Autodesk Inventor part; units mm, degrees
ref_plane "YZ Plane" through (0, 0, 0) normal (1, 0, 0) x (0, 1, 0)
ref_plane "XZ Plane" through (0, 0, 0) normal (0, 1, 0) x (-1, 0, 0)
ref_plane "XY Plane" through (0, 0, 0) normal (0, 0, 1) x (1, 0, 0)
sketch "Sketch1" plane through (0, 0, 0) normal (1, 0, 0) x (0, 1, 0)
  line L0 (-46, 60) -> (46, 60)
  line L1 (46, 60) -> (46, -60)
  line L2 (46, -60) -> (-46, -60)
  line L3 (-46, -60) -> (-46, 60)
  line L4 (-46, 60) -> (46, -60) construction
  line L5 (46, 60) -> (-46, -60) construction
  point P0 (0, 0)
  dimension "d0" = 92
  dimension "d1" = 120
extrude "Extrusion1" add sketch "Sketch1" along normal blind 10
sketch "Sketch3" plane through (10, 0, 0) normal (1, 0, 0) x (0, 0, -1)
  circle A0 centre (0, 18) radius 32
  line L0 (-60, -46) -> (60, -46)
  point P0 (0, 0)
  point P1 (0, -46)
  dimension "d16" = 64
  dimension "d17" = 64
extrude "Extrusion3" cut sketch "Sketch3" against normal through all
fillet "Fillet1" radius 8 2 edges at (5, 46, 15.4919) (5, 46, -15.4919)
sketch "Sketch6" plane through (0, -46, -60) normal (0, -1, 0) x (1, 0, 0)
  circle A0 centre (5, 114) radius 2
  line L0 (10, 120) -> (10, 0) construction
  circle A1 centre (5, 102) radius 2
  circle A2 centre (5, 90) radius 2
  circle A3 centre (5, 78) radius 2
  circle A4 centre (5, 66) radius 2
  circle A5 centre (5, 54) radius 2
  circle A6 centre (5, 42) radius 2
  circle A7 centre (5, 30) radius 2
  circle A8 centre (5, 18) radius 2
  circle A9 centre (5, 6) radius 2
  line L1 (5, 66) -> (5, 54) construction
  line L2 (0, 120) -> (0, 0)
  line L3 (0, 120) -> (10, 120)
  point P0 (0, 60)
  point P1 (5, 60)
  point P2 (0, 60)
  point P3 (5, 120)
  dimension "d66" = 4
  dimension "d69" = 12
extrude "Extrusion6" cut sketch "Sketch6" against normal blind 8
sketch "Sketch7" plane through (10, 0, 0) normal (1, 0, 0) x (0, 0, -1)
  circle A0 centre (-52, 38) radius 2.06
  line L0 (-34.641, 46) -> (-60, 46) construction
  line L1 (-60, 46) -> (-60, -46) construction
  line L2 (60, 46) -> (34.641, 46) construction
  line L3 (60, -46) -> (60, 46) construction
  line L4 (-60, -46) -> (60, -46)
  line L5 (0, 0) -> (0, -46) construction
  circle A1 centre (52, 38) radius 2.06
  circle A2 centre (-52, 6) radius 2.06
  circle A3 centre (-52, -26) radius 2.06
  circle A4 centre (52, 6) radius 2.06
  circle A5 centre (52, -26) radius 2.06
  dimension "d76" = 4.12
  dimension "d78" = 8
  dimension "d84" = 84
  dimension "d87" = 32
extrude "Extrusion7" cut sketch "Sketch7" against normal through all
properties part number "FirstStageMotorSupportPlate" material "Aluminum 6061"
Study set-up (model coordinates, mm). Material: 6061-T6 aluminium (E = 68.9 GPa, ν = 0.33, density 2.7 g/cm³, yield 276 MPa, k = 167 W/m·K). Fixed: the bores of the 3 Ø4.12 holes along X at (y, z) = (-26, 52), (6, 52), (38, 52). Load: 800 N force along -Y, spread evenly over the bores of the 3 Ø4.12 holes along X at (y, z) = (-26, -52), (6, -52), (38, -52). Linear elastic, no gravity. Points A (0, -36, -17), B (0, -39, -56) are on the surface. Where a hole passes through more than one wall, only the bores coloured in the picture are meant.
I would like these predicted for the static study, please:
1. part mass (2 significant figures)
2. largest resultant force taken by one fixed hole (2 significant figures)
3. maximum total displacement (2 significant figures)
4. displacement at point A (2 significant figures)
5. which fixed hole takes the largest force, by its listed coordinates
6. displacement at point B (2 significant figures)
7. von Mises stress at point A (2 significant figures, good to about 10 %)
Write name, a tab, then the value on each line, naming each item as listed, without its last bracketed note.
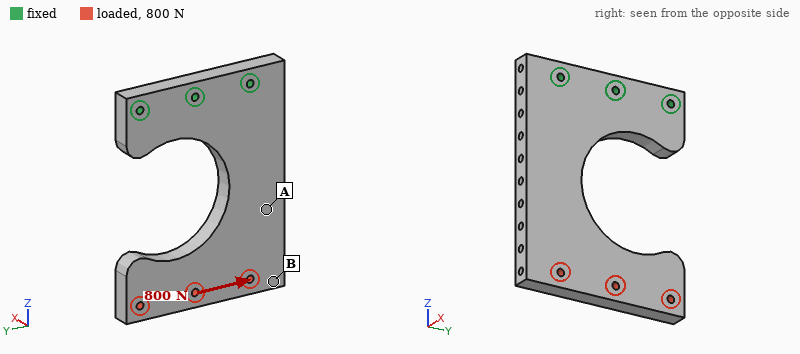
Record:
part mass	210 g
largest resultant force taken by one fixed hole	2.1 kN
maximum total displacement	0.17 mm
displacement at point A	0.055 mm
which fixed hole takes the largest force, by its listed coordinates	(-26, 52)
displacement at point B	0.12 mm
von Mises stress at point A	8.9 MPa
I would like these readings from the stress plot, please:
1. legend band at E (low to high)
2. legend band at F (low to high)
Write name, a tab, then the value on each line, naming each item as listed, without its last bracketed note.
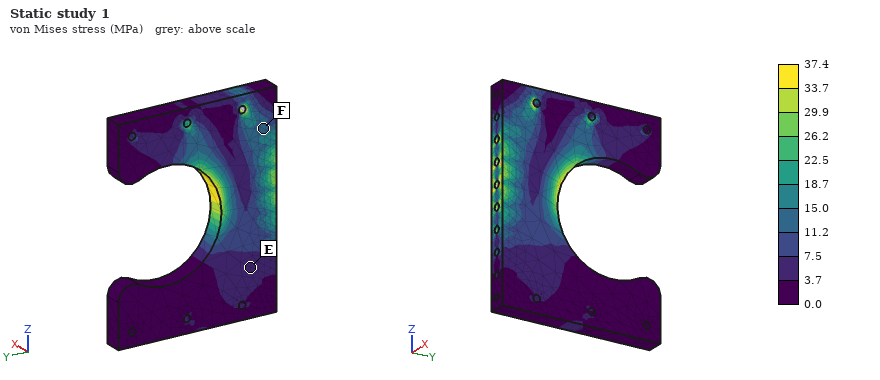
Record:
legend band at E	3.7 to 7.5 MPa
legend band at F	11.2 to 15.0 MPa
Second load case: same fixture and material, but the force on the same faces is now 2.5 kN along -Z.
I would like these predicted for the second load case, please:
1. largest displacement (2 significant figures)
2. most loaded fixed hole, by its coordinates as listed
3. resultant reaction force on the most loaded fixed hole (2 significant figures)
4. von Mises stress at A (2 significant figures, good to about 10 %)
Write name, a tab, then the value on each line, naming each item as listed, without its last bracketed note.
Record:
largest displacement	0.32 mm
most loaded fixed hole, by its coordinates as listed	(6, 52)
resultant reaction force on the most loaded fixed hole	2.1 kN
von Mises stress at A	14 MPa
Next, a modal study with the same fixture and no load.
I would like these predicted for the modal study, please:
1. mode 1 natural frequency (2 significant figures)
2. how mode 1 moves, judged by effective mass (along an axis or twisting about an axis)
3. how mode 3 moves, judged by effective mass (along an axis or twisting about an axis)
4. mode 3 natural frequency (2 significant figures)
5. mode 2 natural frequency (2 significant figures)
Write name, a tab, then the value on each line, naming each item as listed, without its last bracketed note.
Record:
mode 1 natural frequency	440 Hz
how mode 1 moves, judged by effective mass	along X
how mode 3 moves, judged by effective mass	along Y
mode 3 natural frequency	1400 Hz
mode 2 natural frequency	1100 Hz
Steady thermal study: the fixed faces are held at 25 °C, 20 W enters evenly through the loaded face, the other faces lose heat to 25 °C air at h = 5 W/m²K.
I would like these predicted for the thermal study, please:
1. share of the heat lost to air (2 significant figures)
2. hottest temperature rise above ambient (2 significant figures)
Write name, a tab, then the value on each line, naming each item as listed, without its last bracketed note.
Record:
share of the heat lost to air	8.9 %
hottest temperature rise above ambient	39 K
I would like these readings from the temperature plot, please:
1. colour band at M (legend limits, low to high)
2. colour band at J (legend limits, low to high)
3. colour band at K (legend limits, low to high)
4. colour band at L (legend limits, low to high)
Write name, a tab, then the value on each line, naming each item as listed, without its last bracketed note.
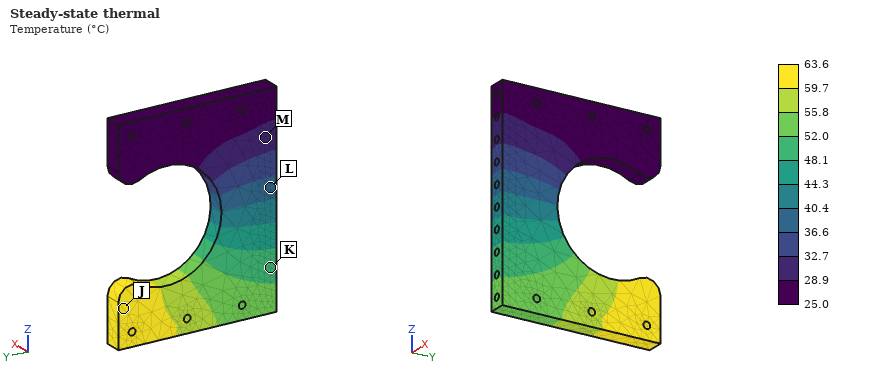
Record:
colour band at M	28.9 to 32.7 °C
colour band at J	59.7 to 63.6 °C
colour band at K	48.1 to 52.0 °C
colour band at L	36.6 to 40.4 °C
